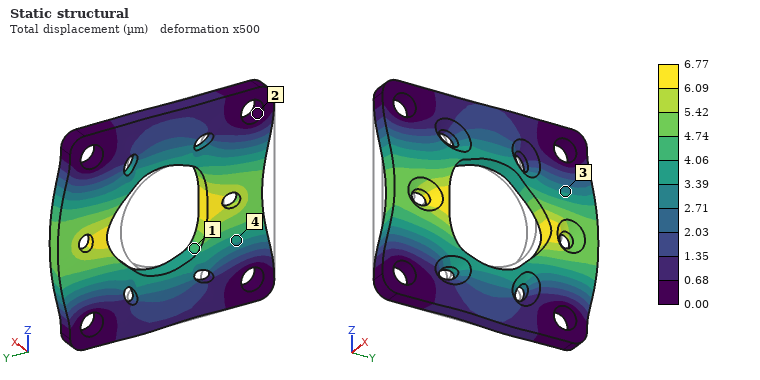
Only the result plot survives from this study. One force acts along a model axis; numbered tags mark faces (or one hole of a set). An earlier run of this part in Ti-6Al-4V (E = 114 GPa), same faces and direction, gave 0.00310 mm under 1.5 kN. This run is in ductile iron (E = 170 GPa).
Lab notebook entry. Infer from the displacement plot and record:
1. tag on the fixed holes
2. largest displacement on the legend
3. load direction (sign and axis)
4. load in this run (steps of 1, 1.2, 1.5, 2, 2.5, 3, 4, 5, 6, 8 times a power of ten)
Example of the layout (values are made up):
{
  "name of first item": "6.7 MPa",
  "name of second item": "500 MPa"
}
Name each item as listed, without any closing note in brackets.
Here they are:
{
  "tag on the fixed holes": "2",
  "largest displacement on the legend": "6.77 µm",
  "load direction": "+Y",
  "load in this run": "5 kN"
}
